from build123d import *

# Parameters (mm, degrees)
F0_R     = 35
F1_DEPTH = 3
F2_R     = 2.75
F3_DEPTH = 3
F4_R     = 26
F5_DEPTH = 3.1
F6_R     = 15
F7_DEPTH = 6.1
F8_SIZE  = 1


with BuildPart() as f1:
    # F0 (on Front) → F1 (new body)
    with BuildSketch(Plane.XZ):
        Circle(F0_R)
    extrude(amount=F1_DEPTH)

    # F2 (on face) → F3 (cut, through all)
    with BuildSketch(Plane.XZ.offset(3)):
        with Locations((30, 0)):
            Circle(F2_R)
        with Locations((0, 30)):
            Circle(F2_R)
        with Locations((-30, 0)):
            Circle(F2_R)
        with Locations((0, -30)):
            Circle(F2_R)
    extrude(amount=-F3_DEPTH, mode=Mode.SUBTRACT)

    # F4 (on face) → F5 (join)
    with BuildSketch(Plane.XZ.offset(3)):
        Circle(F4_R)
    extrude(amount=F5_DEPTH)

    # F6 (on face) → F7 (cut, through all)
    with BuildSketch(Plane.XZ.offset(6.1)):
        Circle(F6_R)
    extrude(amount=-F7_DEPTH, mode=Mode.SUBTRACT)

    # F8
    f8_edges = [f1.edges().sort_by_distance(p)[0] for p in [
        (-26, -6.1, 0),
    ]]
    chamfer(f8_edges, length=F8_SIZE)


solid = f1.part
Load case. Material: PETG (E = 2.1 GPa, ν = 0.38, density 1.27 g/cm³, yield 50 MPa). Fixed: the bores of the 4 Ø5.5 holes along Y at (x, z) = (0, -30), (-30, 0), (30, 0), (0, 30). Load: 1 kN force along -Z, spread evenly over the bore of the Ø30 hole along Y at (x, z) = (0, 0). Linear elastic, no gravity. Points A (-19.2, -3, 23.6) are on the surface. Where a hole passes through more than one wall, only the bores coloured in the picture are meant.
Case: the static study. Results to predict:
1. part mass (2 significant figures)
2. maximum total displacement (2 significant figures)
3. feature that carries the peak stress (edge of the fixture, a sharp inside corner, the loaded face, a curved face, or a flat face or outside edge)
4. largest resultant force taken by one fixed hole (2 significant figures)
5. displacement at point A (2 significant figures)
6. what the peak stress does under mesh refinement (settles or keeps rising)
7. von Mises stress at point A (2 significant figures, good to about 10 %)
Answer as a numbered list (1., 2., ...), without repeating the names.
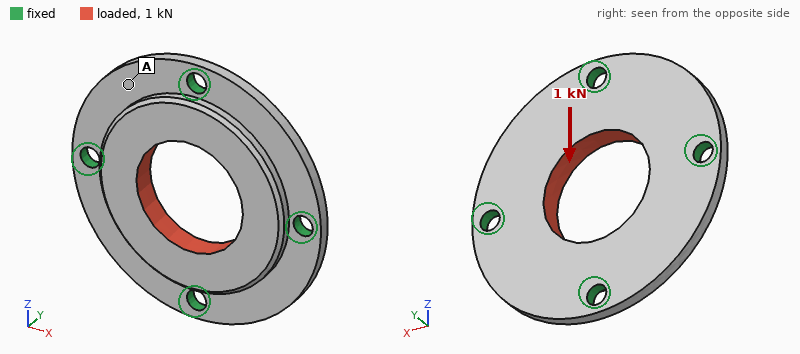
1. 17 g
2. 55 µm
3. edge of the fixture
4. 280 N
5. 36 µm
6. keeps rising
7. 1.6 MPa
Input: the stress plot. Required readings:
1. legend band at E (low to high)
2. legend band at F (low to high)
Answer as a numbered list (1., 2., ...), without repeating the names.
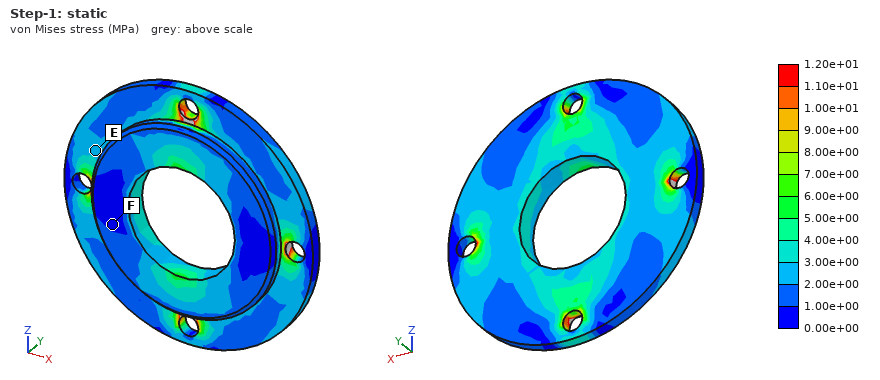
1. 2.00e+00 to 3.00e+00 MPa
2. 0.00e+00 to 1.00e+00 MPa
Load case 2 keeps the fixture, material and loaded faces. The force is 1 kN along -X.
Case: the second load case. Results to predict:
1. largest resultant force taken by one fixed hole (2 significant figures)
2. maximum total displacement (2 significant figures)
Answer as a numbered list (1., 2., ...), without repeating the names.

1. 280 N
2. 54 µm
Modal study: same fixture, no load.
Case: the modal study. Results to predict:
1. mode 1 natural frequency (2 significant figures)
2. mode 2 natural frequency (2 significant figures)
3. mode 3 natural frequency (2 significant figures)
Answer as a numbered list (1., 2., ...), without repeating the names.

1. 2500 Hz
2. 2800 Hz
3. 2800 Hz
